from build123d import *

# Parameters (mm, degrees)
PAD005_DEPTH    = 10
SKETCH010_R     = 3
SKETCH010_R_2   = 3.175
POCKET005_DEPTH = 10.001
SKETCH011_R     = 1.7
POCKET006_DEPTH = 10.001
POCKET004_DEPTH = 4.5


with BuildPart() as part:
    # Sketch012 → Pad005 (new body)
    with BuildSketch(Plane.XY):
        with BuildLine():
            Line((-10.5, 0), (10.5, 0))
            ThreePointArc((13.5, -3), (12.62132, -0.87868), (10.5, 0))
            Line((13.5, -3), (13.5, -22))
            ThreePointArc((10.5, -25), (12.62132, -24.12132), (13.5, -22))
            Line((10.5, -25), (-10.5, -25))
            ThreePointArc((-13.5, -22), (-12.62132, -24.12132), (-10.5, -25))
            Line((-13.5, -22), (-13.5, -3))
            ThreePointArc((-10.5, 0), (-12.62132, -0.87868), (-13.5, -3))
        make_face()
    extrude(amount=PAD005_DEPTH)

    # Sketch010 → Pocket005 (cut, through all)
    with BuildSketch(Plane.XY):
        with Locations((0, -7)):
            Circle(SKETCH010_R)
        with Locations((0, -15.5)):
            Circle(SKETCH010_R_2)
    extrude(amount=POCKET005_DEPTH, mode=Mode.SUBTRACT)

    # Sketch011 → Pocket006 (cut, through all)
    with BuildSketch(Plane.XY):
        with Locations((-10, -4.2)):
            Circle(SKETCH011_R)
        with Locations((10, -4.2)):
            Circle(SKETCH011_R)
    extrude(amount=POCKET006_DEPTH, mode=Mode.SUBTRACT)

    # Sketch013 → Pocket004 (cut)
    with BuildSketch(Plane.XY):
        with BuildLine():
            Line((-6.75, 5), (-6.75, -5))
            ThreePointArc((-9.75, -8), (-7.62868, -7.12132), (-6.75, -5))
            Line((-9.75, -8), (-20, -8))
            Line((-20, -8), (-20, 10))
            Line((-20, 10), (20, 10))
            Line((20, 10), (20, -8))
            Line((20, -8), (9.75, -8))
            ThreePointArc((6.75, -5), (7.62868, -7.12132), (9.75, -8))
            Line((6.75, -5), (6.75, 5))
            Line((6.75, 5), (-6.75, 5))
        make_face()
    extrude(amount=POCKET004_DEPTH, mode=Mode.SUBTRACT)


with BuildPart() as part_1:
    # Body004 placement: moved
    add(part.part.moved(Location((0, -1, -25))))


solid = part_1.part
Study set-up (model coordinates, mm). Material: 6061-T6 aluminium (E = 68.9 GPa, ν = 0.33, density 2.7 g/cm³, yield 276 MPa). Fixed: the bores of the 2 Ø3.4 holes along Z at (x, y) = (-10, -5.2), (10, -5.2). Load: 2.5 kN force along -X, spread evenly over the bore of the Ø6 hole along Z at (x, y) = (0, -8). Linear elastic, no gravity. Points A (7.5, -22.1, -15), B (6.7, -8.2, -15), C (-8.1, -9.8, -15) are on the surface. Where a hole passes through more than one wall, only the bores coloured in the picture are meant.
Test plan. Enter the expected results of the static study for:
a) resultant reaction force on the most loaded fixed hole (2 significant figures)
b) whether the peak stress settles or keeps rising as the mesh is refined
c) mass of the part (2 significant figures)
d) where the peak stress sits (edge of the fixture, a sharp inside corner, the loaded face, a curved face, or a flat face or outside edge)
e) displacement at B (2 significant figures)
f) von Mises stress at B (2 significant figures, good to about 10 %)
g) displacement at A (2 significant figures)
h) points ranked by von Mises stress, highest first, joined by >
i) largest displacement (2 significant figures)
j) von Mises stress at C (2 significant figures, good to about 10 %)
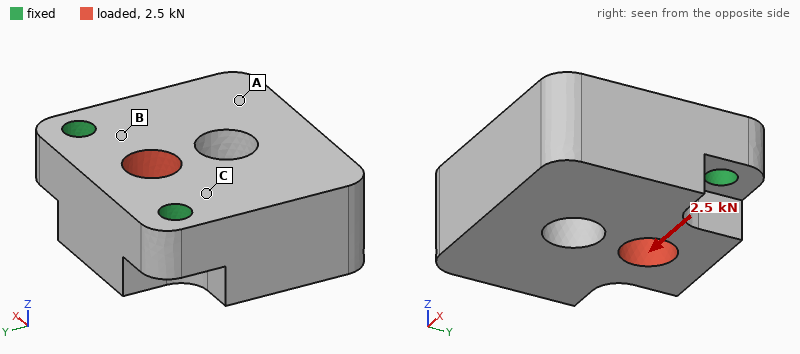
1.3 kN
keeps rising
15 g
edge of the fixture
1.7 µm
20 MPa
3.5 µm
B > C > A
4.7 µm
11 MPa
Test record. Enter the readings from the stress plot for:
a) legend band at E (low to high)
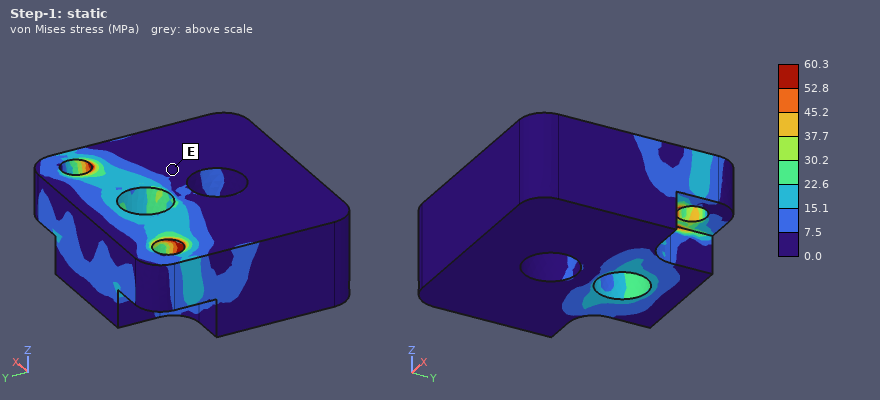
0.0 to 7.5 MPa
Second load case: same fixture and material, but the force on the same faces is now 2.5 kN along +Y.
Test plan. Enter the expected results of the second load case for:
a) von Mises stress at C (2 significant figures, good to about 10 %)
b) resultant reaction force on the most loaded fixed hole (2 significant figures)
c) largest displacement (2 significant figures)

11 MPa
1.3 kN
21 µm
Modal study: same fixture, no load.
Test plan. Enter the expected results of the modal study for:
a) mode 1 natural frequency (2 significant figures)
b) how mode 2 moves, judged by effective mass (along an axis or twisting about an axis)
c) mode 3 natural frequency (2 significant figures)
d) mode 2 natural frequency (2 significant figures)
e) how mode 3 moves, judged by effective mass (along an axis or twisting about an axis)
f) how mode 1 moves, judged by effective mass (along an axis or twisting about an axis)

8300 Hz
along X
22 kHz
20 kHz
along X
along Z
